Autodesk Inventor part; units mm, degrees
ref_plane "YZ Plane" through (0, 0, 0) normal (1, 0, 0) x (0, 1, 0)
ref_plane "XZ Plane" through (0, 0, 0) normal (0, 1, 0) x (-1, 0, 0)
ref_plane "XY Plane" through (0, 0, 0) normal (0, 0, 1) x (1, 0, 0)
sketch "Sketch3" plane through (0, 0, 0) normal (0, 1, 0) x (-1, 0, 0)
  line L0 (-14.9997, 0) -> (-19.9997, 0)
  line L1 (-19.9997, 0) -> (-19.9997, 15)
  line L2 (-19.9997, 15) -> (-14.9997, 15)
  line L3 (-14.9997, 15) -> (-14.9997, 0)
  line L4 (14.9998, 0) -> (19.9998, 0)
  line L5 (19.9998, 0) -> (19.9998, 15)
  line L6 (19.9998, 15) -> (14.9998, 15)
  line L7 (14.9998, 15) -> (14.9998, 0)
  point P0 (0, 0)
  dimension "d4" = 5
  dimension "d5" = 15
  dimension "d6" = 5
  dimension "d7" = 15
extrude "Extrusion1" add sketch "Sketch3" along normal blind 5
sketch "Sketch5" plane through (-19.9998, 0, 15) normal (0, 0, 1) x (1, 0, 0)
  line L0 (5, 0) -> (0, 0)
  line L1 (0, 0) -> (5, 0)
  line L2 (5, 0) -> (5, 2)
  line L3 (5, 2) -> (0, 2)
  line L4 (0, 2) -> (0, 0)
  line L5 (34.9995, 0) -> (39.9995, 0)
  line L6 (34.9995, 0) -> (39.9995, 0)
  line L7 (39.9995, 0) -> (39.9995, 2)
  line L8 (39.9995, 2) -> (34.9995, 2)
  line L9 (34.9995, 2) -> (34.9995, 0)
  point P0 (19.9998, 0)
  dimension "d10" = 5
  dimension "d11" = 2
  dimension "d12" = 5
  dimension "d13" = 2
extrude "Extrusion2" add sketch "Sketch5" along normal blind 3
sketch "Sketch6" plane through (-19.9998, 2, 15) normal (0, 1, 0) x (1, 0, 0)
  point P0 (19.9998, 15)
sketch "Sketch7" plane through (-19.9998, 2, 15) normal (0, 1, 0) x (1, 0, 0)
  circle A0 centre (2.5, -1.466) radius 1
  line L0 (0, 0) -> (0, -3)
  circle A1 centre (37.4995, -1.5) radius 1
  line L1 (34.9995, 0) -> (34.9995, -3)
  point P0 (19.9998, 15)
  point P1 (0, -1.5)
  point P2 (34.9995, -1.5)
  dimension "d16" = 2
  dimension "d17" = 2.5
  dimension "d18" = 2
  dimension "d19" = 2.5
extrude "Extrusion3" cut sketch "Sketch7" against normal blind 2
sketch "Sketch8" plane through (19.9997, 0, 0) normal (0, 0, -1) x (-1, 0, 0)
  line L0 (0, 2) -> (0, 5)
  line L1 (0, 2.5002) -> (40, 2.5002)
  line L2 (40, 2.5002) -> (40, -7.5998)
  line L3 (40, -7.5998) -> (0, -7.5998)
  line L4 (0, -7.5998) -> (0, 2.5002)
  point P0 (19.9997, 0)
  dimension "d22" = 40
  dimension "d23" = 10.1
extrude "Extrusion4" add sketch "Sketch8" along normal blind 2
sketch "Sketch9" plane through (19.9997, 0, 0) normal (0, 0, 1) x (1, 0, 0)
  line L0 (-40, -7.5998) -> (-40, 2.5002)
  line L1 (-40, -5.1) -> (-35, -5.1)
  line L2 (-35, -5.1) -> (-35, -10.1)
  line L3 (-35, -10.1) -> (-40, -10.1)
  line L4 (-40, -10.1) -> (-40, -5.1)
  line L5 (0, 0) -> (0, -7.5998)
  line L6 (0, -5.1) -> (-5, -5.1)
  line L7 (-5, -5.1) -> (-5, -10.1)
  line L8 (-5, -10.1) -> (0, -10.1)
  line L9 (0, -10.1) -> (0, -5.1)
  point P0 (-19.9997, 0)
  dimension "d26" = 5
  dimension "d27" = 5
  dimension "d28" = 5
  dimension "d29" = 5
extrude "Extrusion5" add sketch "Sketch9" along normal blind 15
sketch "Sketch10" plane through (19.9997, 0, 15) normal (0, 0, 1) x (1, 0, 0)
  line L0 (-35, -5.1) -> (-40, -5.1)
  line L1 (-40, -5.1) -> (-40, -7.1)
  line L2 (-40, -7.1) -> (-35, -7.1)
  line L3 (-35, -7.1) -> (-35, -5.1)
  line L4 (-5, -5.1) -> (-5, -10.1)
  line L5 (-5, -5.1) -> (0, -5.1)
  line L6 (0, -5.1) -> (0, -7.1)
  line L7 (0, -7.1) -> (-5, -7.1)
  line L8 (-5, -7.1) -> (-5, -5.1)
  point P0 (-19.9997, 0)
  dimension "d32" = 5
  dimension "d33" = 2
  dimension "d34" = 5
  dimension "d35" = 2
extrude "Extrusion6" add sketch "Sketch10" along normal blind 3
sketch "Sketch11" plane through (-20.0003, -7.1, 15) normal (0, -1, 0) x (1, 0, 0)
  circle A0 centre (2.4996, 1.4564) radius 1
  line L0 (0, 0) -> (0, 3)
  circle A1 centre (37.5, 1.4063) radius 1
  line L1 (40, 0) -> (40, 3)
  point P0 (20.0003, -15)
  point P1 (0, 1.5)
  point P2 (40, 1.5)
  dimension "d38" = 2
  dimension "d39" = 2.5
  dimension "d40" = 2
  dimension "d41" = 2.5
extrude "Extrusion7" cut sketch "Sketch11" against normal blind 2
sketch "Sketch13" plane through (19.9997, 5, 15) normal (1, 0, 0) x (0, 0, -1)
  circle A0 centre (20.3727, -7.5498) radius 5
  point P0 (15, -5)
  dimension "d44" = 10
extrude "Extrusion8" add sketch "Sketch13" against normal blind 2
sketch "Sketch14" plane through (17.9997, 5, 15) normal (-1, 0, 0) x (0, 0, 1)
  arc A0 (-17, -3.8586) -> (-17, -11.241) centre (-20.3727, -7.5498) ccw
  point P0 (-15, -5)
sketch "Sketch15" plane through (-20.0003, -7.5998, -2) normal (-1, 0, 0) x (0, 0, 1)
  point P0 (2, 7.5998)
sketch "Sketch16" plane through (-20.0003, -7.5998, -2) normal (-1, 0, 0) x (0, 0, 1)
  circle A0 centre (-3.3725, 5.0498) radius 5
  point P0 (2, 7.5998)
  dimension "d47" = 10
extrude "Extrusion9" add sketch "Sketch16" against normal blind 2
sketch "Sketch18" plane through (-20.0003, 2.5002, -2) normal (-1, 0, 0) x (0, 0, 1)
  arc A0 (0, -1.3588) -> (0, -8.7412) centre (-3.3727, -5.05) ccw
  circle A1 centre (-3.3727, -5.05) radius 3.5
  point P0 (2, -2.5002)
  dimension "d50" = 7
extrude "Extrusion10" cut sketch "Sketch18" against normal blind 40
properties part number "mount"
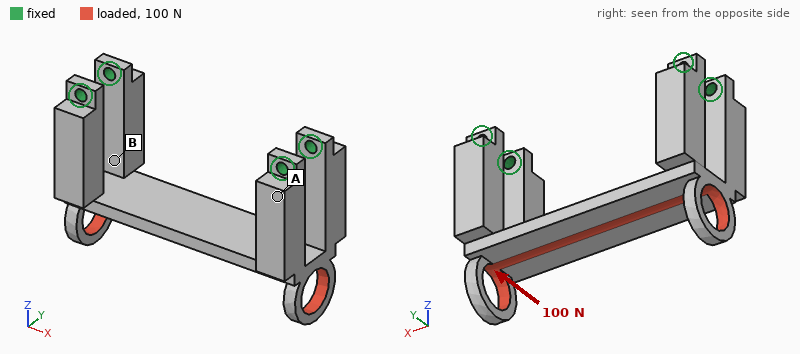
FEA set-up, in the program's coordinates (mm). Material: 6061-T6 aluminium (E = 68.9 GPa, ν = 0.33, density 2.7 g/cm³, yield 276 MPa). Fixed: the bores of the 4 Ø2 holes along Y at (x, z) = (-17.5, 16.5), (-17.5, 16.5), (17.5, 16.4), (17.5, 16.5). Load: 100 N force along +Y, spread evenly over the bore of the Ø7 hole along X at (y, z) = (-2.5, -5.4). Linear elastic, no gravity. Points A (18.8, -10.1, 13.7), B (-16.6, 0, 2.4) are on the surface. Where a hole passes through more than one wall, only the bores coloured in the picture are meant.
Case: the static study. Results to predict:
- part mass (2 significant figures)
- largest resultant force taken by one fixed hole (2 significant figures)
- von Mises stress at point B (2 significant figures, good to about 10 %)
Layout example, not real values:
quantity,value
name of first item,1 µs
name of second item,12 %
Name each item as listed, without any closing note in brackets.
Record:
quantity,value
part mass,6.8 g
largest resultant force taken by one fixed hole,76 N
von Mises stress at point B,16 MPa
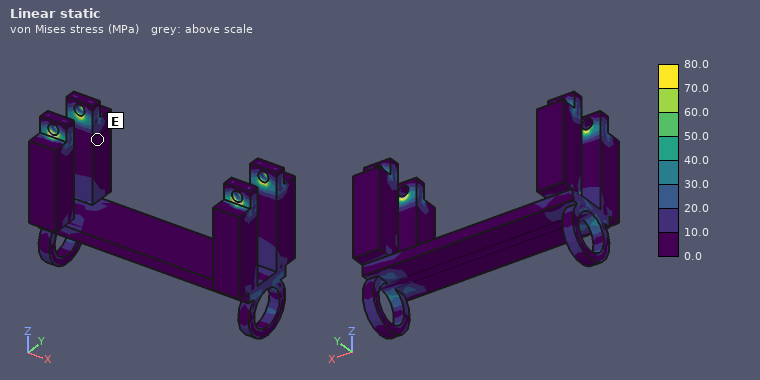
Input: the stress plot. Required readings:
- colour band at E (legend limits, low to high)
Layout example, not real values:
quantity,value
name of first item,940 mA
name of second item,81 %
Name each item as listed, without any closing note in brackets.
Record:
quantity,value
colour band at E,0.0 to 10.0 MPa
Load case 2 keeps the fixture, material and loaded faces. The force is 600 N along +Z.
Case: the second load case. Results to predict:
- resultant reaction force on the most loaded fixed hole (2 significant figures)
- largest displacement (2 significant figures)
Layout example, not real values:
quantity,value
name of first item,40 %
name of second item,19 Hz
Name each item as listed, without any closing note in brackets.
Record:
quantity,value
resultant reaction force on the most loaded fixed hole,150 N
largest displacement,56 µm
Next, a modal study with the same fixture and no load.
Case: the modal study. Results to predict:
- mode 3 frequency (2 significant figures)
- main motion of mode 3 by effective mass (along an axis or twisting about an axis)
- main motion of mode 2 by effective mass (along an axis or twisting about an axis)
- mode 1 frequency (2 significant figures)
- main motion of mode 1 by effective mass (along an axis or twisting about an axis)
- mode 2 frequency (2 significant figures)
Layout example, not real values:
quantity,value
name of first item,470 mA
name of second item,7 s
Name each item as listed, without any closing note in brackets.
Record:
quantity,value
mode 3 frequency,6500 Hz
main motion of mode 3 by effective mass,twisting about Z
main motion of mode 2 by effective mass,along X
mode 1 frequency,4800 Hz
main motion of mode 1 by effective mass,along Y
mode 2 frequency,5200 Hz
